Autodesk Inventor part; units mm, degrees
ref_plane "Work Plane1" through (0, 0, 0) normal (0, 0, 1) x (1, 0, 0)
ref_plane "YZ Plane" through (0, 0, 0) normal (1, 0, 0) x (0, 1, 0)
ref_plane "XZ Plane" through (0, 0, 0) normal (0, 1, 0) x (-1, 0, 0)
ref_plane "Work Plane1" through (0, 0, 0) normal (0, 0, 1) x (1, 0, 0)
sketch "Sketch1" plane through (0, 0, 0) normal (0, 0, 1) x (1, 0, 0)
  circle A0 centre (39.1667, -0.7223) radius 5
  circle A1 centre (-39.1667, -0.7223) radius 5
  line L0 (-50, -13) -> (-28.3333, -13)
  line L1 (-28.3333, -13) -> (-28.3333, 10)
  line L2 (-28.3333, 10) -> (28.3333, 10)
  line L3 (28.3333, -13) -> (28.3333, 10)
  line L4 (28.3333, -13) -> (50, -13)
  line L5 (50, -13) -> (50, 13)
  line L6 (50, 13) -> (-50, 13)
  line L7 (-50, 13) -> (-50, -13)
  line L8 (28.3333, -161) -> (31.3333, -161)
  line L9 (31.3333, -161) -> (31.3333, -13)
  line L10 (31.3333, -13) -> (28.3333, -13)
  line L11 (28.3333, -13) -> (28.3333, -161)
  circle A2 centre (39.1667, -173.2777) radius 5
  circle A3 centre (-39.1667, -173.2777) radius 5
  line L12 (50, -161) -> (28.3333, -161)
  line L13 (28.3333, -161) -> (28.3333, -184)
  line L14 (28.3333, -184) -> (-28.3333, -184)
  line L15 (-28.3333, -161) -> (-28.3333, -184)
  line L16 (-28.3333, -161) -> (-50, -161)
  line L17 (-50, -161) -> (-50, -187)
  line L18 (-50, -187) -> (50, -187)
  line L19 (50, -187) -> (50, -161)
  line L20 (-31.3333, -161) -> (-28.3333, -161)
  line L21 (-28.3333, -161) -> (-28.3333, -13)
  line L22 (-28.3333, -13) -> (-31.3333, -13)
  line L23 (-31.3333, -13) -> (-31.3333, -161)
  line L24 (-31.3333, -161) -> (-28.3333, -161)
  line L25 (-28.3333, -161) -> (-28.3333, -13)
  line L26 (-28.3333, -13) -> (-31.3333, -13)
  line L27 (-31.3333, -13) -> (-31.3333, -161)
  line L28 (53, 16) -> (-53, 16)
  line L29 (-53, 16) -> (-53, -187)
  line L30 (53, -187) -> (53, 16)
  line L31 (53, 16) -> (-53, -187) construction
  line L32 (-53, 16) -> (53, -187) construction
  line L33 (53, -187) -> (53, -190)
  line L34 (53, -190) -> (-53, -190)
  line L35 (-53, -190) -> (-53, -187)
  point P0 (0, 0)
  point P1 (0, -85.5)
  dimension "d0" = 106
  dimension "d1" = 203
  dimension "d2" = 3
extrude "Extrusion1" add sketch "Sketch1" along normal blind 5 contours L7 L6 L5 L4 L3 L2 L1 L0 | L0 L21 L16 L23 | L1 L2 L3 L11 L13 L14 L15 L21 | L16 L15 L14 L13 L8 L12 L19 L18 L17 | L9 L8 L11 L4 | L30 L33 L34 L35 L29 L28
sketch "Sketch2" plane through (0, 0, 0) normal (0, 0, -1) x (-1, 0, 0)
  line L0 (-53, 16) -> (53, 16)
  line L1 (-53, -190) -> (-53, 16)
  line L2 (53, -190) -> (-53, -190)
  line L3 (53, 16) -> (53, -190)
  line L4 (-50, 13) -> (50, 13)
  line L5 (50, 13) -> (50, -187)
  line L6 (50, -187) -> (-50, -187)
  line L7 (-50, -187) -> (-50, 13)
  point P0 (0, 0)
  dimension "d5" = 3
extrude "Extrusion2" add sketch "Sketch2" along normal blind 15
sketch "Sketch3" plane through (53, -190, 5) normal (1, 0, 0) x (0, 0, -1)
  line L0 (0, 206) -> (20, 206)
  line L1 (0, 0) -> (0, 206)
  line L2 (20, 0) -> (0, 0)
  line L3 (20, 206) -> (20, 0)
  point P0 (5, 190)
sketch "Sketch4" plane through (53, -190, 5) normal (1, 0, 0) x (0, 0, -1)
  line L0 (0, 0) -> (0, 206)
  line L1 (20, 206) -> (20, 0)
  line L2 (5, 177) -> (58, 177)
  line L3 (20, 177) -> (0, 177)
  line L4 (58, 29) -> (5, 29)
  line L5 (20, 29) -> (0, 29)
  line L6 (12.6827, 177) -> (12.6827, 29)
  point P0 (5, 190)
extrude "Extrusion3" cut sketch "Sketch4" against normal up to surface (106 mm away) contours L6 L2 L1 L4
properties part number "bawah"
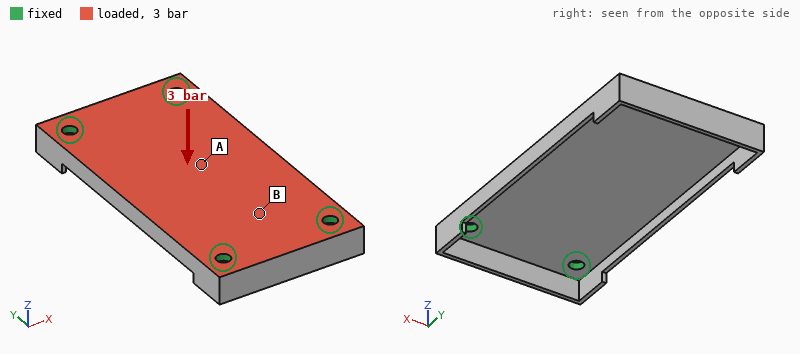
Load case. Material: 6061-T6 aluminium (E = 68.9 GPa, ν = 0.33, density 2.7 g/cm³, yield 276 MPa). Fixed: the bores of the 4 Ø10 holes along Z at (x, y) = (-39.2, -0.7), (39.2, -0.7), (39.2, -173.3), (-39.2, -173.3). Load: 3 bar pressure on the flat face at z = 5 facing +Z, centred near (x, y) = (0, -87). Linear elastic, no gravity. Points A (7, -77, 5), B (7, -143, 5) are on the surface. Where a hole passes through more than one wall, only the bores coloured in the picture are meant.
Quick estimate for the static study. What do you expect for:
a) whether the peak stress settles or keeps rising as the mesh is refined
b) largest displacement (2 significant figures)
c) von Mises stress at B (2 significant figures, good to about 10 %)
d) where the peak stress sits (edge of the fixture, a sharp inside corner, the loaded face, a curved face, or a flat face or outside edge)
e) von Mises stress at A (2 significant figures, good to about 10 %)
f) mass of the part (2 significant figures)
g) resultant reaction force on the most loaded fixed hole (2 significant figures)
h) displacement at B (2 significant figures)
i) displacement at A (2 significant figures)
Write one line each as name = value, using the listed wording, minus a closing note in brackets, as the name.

whether the peak stress settles or keeps rising as the mesh is refined = keeps rising
largest displacement = 0.56 mm
von Mises stress at B = 23 MPa
where the peak stress sits = edge of the fixture
von Mises stress at A = 52 MPa
mass of the part = 350 g
resultant reaction force on the most loaded fixed hole = 1.6 kN
displacement at B = 0.26 mm
displacement at A = 0.55 mm
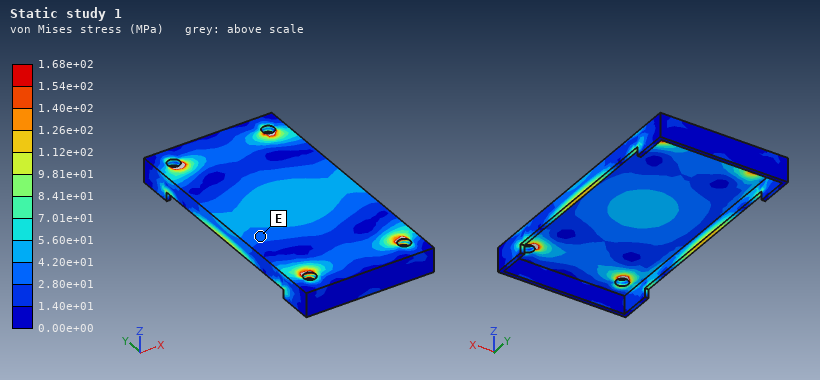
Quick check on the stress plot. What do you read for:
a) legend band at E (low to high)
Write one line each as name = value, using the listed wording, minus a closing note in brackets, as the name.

legend band at E = 2.80e+01 to 4.20e+01 MPa
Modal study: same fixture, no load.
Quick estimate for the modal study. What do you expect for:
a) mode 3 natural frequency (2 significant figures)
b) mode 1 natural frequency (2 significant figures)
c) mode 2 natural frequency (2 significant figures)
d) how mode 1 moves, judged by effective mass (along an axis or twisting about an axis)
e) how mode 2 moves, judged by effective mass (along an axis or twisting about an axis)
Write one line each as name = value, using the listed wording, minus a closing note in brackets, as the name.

mode 3 natural frequency = 2800 Hz
mode 1 natural frequency = 1200 Hz
mode 2 natural frequency = 1700 Hz
how mode 1 moves, judged by effective mass = along Z
how mode 2 moves, judged by effective mass = twisting about Y
